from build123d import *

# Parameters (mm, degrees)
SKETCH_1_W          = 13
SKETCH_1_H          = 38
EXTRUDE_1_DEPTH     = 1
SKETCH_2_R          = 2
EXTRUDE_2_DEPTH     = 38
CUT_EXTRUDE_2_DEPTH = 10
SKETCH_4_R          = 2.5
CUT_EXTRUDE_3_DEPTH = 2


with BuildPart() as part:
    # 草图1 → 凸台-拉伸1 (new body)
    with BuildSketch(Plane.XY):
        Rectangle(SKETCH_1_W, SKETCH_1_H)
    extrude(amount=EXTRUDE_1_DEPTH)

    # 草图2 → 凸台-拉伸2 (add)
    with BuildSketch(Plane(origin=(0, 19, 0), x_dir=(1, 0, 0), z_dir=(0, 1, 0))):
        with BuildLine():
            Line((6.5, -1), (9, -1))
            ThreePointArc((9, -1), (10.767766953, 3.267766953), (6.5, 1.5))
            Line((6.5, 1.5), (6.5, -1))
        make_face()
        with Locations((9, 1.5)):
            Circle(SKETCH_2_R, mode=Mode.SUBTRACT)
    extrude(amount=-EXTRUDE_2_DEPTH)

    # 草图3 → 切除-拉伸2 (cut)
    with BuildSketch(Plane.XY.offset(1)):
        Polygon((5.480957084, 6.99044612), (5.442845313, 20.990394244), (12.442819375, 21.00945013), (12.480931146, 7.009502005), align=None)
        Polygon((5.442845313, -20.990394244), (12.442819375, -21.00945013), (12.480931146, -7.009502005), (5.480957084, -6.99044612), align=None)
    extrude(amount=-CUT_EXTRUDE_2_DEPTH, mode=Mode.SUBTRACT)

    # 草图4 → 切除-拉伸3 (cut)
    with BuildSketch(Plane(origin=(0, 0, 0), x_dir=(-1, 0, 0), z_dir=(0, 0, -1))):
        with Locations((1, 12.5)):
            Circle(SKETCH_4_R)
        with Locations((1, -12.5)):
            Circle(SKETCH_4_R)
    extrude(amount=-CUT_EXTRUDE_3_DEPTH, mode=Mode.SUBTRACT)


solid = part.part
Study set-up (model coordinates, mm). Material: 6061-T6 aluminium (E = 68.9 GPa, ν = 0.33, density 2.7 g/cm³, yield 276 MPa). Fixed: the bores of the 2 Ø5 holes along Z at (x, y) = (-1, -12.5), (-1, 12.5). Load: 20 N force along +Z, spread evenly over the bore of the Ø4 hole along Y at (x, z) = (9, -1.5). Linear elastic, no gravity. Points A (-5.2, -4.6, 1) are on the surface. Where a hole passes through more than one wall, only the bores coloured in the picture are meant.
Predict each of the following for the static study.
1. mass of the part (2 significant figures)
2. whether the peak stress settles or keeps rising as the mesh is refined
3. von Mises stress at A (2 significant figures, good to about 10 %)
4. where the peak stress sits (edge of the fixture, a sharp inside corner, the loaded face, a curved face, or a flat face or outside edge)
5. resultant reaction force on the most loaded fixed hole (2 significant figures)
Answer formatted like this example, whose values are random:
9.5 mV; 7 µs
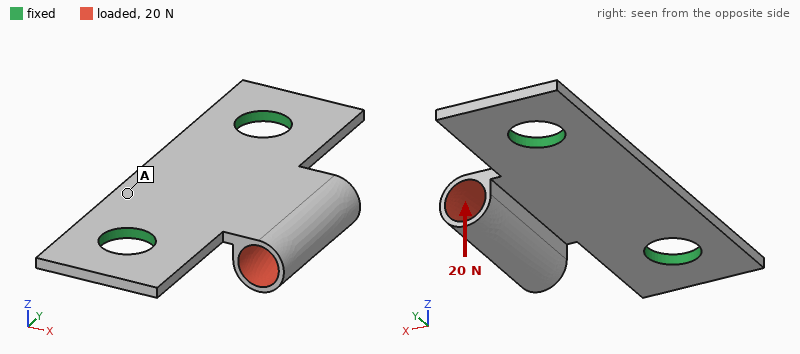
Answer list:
1.5 g; keeps rising; 9.1 MPa; a sharp inside corner; 10 N
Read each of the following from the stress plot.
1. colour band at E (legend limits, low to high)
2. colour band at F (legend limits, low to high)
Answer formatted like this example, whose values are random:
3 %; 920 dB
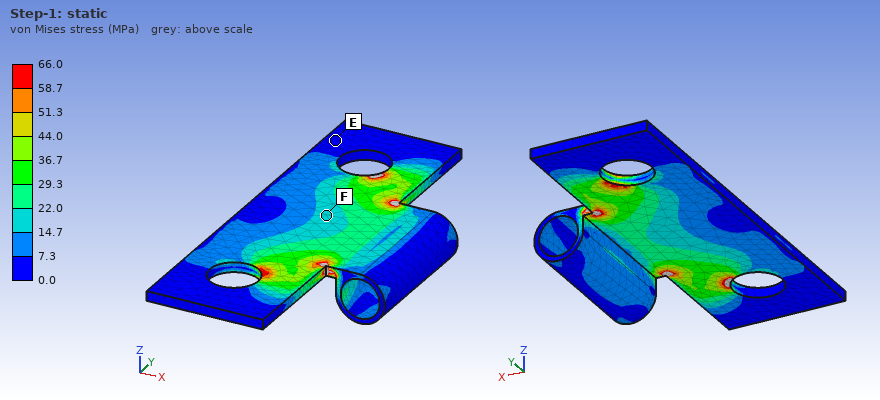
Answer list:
0.0 to 7.3 MPa; 14.7 to 22.0 MPa
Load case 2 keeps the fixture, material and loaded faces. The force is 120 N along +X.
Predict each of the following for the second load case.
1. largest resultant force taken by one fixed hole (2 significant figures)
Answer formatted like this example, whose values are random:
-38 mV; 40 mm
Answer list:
63 N
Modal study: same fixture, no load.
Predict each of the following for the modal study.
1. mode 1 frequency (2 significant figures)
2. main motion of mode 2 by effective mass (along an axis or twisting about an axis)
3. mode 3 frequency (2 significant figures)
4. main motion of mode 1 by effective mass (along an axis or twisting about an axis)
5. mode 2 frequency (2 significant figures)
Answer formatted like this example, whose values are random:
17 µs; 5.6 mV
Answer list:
4700 Hz; along Z; 14 kHz; along Z; 12 kHz
